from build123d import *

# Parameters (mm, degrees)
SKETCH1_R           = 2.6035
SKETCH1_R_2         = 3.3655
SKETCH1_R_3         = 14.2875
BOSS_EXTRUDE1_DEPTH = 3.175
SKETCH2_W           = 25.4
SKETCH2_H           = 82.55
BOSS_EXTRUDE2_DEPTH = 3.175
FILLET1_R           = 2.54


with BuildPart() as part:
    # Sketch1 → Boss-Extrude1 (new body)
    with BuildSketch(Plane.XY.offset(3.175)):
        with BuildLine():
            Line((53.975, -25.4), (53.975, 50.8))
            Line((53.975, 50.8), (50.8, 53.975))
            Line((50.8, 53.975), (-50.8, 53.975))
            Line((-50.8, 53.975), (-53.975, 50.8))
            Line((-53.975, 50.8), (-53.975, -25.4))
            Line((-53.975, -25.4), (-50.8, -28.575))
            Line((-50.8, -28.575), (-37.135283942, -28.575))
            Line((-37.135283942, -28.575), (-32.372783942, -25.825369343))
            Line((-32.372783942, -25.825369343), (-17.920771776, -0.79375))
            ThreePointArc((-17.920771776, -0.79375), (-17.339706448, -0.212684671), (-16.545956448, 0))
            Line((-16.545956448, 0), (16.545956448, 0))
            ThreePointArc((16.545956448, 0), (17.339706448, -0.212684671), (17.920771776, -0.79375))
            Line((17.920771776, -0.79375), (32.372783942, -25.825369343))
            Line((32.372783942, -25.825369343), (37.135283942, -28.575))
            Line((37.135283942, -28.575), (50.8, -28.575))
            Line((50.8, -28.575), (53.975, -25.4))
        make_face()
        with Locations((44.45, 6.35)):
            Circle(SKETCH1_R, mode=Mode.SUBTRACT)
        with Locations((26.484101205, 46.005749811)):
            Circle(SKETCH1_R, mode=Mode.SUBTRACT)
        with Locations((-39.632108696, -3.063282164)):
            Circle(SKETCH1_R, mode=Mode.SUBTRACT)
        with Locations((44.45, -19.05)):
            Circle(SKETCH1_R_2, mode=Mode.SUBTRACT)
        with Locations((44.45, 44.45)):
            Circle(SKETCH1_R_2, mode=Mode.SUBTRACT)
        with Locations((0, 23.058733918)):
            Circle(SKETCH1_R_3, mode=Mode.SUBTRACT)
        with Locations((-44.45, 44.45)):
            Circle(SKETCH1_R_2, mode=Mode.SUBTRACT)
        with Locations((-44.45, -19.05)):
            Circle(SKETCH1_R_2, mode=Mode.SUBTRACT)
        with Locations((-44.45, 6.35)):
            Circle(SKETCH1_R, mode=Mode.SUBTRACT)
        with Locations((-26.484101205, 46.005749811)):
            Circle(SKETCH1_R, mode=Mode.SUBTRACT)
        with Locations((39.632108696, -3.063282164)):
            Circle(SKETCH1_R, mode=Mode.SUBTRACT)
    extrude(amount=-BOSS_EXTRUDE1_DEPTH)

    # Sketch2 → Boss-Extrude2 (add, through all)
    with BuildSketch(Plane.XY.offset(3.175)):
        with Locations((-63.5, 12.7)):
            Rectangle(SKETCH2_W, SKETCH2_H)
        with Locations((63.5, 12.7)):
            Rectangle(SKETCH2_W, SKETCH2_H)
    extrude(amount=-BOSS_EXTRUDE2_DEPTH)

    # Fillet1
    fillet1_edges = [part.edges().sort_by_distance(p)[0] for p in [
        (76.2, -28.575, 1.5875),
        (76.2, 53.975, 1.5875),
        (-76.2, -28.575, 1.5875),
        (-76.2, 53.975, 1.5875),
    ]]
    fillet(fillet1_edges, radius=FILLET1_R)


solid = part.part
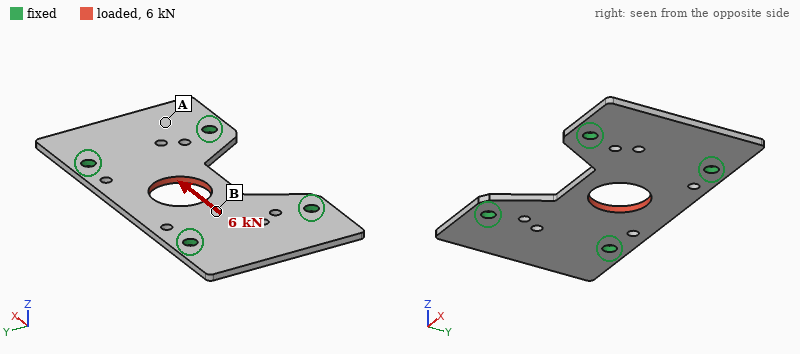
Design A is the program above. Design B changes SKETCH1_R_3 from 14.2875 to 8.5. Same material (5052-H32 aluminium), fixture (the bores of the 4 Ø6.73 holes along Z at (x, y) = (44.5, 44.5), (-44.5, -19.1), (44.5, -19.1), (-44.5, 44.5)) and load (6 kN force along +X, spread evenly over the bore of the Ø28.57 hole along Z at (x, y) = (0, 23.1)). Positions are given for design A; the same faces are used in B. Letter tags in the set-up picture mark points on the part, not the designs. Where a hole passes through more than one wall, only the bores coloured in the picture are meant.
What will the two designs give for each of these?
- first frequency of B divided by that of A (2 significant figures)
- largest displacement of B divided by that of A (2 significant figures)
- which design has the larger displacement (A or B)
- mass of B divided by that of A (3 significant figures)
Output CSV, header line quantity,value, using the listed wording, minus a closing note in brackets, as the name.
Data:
quantity,value
first frequency of B divided by that of A,0.97
largest displacement of B divided by that of A,1.1
which design has the larger displacement,B
mass of B divided by that of A,1.04
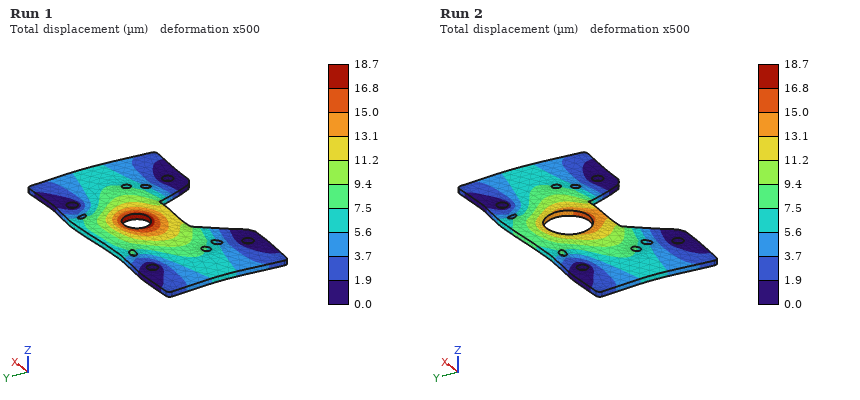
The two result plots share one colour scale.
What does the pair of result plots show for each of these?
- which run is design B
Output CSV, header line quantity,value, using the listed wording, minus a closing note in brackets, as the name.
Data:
quantity,value
which run is design B,Run 1
